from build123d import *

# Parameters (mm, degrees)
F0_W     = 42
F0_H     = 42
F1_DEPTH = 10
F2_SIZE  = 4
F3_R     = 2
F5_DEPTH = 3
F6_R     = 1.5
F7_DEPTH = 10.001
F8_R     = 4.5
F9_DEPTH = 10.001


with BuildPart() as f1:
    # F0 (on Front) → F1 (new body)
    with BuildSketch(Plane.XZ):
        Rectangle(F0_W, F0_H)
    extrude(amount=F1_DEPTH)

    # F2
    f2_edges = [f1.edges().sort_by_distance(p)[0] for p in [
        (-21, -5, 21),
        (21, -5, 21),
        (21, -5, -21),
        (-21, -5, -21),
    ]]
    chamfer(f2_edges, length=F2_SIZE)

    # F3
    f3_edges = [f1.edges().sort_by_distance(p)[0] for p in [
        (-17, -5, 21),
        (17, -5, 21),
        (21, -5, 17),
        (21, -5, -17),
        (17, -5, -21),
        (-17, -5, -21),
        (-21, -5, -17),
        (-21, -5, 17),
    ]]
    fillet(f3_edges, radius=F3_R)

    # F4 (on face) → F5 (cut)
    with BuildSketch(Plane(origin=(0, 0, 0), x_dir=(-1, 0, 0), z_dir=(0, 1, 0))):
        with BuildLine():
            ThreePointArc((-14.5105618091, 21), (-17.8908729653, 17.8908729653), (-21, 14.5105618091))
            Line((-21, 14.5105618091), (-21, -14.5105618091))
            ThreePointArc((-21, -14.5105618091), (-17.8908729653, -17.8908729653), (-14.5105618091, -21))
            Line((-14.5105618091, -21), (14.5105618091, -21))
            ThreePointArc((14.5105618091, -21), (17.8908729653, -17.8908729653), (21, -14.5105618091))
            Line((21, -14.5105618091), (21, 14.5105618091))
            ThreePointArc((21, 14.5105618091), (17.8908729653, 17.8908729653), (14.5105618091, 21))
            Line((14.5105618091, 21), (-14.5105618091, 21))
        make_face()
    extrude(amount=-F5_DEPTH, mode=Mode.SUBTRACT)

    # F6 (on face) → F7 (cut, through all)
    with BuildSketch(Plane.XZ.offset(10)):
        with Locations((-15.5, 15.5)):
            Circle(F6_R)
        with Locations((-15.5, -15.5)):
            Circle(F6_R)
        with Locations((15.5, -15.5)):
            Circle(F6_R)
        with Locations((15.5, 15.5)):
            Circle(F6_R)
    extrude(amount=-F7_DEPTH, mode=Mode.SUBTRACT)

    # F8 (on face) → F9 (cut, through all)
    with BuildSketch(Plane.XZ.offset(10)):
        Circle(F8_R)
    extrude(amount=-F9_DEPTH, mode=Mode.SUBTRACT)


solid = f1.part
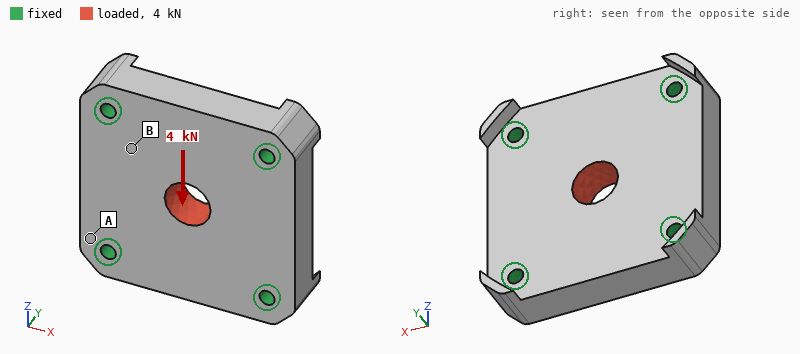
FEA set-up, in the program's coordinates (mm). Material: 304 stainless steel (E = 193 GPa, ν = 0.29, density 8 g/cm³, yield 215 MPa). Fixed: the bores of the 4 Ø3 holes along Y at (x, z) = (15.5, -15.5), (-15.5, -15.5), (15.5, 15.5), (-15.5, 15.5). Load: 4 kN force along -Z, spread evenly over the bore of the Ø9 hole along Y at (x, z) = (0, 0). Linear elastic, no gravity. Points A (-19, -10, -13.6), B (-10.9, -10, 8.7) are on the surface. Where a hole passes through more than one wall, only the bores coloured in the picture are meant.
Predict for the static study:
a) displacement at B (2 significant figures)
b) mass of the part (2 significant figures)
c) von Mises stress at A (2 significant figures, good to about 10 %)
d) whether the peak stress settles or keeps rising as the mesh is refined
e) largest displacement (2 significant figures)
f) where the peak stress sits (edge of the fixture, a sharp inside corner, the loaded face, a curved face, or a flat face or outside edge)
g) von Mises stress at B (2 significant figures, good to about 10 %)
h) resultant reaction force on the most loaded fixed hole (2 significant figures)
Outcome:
0.72 µm
93 g
5.4 MPa
keeps rising
2.0 µm
edge of the fixture
15 MPa
1.1 kN
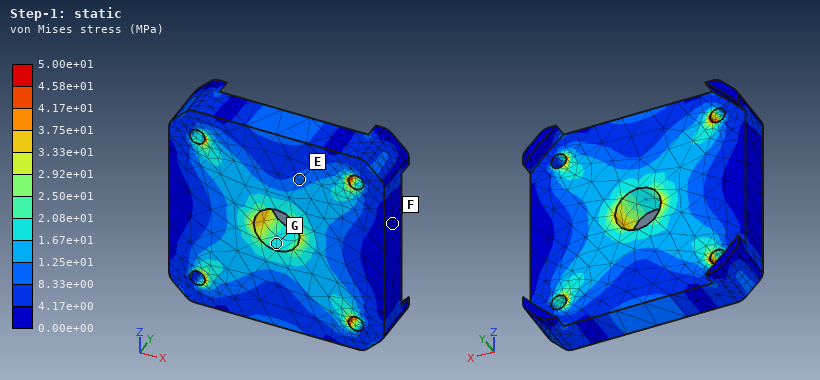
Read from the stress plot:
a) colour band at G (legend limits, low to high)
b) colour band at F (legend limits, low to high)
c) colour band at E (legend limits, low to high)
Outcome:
1.67e+01 to 2.08e+01 MPa
0.00e+00 to 4.17e+00 MPa
8.33e+00 to 1.25e+01 MPa
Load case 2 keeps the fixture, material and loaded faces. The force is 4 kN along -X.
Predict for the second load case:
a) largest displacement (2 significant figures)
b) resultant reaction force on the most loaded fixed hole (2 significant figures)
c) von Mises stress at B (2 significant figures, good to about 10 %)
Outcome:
2.0 µm
1.1 kN
16 MPa
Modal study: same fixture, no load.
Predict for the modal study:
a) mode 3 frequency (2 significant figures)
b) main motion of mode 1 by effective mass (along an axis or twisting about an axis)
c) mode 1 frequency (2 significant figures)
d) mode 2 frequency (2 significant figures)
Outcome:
30 kHz
along Y
20 kHz
30 kHz
